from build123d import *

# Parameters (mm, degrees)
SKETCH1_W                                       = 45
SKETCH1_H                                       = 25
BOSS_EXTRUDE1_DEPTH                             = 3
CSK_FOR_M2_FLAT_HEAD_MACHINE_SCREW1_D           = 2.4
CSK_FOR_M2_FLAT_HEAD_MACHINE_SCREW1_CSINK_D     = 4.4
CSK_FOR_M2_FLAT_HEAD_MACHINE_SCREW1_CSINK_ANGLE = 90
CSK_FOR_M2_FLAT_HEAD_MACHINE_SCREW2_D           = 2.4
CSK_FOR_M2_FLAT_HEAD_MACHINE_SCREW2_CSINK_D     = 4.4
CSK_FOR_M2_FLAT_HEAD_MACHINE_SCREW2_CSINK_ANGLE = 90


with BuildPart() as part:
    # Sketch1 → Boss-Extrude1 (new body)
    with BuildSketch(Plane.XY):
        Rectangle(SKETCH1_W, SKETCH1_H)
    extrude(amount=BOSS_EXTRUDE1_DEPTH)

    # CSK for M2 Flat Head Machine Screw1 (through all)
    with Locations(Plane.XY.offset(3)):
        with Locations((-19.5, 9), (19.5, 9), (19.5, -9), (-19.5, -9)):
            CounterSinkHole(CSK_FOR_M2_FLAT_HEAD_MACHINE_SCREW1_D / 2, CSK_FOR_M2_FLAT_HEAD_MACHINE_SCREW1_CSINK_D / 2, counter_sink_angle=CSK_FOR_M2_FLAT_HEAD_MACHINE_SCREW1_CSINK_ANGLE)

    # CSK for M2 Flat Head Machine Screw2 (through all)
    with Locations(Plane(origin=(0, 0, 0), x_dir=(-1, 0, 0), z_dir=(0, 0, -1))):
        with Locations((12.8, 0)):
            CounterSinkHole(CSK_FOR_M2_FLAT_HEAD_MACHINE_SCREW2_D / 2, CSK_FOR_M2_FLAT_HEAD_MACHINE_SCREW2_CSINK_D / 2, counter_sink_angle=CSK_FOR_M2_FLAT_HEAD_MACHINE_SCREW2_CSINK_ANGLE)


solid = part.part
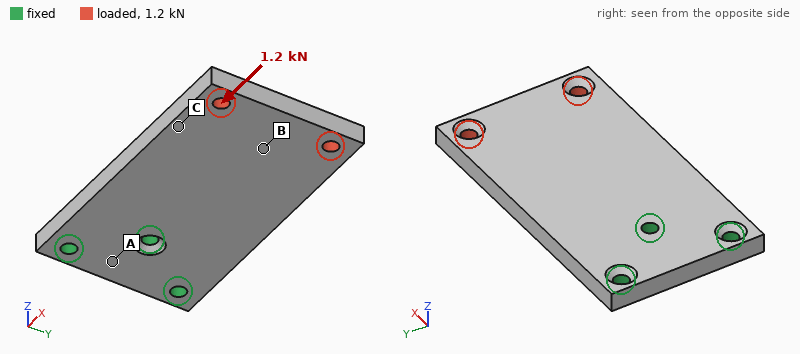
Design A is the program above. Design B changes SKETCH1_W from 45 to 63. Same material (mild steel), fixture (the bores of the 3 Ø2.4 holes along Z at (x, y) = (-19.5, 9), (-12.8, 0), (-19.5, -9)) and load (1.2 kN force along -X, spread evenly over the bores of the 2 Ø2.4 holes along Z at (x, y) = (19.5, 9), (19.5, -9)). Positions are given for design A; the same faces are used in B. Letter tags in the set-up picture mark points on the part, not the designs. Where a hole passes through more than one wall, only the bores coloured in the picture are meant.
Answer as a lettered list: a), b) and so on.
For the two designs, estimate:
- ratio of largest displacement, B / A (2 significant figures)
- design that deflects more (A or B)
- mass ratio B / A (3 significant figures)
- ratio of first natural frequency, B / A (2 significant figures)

a) 1.4
b) B
c) 1.41
d) 0.64
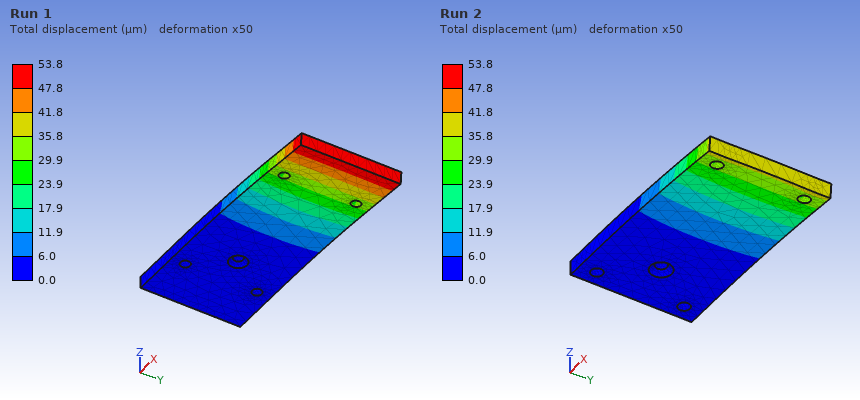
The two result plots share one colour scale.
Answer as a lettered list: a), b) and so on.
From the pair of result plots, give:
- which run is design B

a) Run 1
